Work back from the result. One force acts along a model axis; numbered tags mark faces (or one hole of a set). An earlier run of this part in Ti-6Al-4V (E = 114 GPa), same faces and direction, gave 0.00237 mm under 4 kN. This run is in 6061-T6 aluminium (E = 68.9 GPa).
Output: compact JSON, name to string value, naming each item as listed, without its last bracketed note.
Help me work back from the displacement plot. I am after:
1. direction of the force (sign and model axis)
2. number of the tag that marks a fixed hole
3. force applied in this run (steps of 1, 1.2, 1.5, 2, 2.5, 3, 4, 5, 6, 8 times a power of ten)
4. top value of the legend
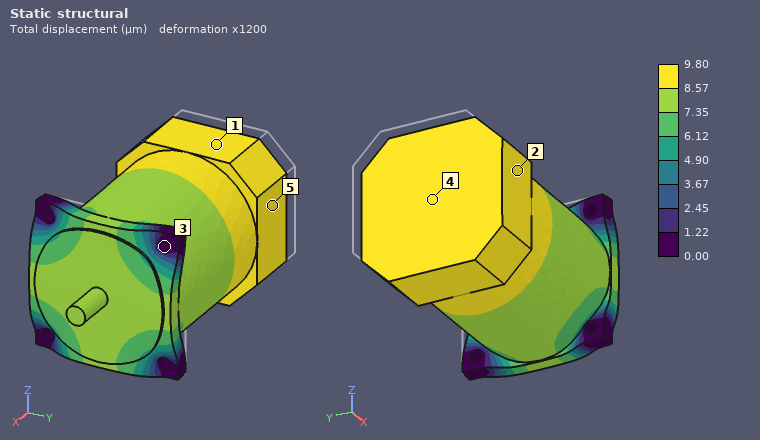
{"direction of the force": "+X", "number of the tag that marks a fixed hole": "3", "force applied in this run": "10 kN", "top value of the legend": "9.80 µm"}
